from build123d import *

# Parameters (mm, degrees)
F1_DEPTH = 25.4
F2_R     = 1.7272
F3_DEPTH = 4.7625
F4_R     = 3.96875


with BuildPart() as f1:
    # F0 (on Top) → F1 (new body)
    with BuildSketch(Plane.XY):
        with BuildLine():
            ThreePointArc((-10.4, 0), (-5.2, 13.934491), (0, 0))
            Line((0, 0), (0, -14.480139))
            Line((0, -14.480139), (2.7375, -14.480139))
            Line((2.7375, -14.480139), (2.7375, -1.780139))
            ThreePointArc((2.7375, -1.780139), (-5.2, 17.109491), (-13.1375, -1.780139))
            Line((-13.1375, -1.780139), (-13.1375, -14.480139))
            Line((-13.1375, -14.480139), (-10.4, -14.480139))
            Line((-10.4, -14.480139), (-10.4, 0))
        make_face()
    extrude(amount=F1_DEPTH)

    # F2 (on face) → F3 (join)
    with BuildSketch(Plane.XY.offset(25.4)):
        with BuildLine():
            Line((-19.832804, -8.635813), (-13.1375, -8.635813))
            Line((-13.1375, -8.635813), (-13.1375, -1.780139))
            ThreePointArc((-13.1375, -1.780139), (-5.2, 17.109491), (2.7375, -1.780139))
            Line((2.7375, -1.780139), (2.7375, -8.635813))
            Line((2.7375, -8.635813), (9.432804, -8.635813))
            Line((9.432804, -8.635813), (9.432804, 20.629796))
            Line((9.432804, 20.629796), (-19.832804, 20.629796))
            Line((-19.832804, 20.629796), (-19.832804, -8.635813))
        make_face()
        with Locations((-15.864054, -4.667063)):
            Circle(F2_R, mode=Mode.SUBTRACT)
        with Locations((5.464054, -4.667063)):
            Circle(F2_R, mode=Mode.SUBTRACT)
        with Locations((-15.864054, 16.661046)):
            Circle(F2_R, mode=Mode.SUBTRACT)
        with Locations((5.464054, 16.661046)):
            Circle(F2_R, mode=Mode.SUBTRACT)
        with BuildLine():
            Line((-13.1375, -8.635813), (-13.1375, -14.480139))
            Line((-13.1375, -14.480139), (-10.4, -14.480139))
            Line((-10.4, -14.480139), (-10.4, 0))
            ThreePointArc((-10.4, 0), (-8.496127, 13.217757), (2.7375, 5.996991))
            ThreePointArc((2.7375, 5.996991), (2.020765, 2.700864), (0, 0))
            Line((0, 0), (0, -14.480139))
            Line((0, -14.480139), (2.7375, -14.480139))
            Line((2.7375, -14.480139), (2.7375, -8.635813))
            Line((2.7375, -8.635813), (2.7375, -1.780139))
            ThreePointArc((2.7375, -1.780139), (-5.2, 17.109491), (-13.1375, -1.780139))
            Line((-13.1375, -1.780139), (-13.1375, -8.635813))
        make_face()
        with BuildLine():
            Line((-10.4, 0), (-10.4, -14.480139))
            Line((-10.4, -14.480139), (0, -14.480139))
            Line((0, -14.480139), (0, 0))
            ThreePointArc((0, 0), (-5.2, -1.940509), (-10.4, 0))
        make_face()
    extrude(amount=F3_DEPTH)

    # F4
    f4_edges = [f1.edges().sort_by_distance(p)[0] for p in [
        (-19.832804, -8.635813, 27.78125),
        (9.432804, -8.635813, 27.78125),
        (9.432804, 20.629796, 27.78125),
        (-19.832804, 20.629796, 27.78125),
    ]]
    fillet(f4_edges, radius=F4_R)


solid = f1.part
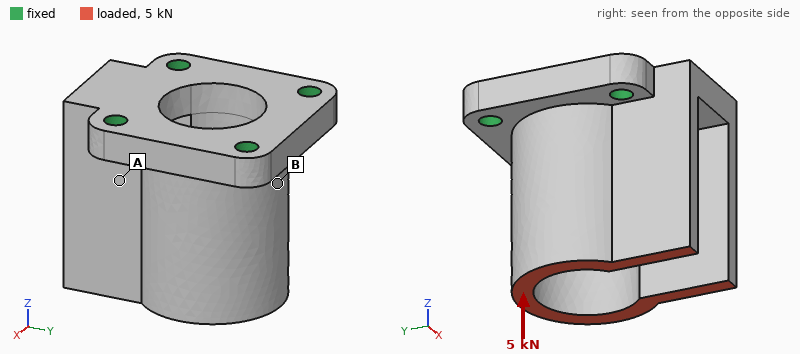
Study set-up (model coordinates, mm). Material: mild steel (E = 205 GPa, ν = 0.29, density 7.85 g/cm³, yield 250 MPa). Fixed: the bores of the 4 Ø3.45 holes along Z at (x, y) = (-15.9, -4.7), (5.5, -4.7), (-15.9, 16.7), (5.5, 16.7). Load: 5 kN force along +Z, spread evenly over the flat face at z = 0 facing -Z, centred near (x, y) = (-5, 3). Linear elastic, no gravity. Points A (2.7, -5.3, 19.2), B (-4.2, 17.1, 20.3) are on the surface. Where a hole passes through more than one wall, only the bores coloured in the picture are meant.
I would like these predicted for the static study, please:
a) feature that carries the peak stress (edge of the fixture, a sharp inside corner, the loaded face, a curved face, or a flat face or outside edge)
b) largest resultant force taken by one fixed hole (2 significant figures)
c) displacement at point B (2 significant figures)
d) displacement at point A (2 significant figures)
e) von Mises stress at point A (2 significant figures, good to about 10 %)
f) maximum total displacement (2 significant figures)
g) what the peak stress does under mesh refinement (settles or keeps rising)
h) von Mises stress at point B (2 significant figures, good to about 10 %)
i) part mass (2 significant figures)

edge of the fixture
1.5 kN
3.0 µm
3.2 µm
34 MPa
5.8 µm
keeps rising
17 MPa
70 g
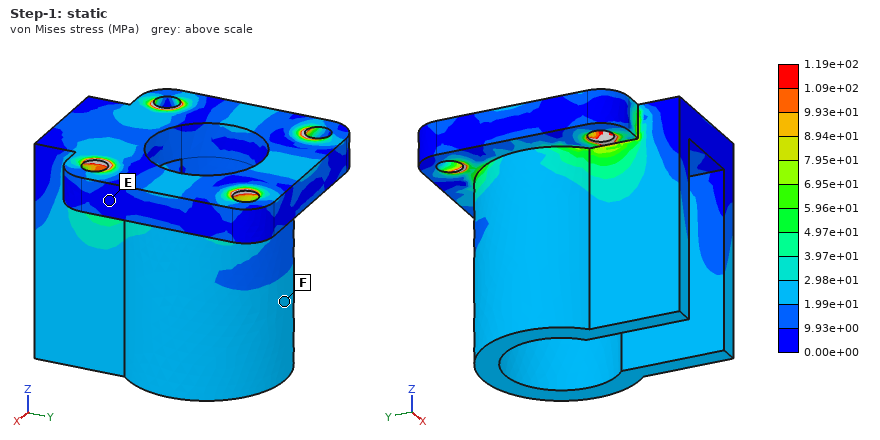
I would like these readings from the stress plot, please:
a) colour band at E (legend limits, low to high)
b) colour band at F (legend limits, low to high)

0.00e+00 to 9.93e+00 MPa
1.99e+01 to 2.98e+01 MPa
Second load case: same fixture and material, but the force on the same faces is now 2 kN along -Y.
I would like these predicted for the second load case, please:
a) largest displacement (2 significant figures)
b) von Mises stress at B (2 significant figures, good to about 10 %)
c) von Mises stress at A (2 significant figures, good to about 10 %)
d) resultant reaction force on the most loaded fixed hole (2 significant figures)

31 µm
40 MPa
41 MPa
1.4 kN
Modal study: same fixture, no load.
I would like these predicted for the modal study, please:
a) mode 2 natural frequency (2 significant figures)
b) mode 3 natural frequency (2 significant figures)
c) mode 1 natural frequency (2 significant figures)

6100 Hz
12 kHz
5900 Hz
